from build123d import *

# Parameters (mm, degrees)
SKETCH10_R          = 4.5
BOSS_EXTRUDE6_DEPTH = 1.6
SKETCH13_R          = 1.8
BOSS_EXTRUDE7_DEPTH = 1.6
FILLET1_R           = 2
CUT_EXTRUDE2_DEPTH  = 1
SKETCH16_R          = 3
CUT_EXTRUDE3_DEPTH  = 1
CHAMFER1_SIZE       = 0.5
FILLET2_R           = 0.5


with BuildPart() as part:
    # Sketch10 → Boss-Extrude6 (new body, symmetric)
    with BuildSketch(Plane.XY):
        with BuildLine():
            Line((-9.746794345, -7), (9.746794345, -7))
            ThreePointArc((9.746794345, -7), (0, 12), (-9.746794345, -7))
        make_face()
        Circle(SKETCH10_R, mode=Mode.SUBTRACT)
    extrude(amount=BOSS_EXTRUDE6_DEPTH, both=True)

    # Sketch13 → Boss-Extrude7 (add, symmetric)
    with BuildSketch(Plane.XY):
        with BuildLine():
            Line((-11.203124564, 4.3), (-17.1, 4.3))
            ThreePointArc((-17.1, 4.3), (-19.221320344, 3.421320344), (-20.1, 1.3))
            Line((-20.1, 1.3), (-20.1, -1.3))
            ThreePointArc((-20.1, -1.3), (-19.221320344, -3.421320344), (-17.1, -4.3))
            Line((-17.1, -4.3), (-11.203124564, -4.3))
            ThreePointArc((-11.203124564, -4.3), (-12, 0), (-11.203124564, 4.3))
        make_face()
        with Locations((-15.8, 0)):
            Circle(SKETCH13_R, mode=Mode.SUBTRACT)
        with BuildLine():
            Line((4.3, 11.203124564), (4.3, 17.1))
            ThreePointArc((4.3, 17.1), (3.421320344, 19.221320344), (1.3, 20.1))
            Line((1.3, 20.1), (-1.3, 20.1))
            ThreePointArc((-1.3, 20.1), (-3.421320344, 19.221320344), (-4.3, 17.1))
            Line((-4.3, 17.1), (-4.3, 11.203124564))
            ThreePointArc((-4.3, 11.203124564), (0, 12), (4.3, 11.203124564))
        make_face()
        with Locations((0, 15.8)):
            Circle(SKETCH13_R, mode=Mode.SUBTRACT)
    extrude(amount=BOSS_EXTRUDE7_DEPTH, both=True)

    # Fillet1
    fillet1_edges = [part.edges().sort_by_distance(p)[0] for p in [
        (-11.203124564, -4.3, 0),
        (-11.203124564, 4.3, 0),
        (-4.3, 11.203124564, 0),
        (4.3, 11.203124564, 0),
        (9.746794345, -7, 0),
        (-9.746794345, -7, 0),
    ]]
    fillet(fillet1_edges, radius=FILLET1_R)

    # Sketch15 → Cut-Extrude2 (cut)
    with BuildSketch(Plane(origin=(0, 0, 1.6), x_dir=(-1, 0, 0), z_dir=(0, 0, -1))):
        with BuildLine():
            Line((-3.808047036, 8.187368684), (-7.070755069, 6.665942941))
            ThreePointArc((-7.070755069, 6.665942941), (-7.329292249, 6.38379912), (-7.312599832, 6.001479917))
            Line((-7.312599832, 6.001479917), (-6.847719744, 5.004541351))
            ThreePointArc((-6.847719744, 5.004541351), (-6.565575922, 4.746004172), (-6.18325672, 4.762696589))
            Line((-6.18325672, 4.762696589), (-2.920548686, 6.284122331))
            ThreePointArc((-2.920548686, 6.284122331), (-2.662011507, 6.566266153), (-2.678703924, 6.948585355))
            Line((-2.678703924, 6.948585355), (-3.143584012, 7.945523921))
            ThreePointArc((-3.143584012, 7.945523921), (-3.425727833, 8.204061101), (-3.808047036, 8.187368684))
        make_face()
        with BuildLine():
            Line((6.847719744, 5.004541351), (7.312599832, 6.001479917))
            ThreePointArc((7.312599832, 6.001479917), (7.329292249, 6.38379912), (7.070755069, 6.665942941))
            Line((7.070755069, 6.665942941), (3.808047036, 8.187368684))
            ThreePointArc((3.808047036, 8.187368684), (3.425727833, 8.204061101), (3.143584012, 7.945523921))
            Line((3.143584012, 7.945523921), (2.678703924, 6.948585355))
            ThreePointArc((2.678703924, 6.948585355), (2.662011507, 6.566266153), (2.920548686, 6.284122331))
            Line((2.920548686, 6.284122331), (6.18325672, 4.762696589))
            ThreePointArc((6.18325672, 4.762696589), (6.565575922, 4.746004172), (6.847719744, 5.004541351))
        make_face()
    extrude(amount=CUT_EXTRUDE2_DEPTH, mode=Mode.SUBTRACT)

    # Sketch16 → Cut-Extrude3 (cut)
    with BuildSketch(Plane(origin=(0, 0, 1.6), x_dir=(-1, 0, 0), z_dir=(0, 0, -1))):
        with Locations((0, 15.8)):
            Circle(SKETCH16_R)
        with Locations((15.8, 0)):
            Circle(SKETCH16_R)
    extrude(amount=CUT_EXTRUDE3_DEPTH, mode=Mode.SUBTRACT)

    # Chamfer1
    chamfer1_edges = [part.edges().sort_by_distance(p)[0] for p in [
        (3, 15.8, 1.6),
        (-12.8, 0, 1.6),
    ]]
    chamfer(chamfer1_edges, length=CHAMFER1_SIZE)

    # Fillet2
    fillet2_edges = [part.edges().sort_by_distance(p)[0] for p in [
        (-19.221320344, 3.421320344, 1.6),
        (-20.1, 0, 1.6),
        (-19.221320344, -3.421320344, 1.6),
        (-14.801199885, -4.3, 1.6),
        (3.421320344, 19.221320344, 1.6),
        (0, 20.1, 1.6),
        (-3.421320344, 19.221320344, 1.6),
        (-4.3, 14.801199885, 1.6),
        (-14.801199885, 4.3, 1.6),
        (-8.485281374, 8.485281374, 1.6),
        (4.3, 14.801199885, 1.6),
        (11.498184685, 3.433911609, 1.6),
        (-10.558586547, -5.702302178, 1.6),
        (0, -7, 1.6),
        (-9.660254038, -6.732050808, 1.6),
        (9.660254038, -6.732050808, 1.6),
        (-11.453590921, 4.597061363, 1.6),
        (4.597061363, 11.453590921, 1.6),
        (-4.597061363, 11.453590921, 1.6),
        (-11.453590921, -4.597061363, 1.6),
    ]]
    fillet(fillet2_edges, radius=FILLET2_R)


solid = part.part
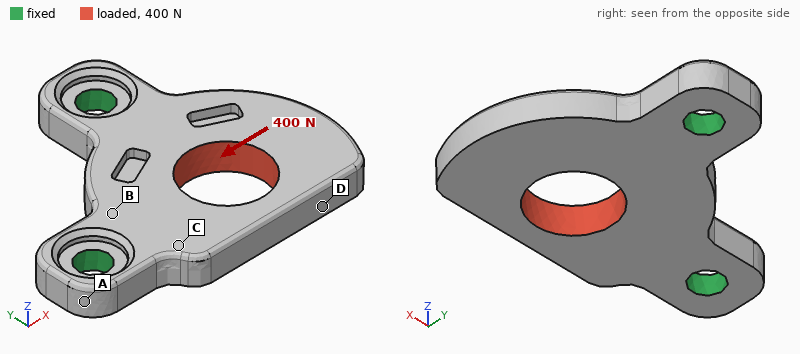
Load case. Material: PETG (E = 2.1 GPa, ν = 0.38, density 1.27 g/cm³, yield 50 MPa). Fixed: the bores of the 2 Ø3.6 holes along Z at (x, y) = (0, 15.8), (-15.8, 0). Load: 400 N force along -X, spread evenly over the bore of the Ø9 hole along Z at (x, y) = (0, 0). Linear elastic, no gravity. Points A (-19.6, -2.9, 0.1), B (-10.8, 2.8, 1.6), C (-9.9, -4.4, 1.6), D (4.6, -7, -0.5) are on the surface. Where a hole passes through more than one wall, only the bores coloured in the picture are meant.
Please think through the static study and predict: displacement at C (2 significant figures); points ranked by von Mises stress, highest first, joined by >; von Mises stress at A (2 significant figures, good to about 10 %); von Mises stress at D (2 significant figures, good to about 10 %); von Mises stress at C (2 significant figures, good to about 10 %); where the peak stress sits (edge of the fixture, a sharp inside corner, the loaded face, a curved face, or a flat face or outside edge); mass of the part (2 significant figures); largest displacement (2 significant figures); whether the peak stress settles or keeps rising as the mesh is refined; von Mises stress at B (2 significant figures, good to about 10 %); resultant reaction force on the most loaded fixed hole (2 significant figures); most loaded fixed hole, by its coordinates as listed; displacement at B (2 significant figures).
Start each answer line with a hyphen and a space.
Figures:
- 0.087 mm
- C > D > B > A
- 2.9 MPa
- 10 MPa
- 13 MPa
- edge of the fixture
- 1.7 g
- 0.22 mm
- keeps rising
- 6.1 MPa
- 340 N
- (-15.8, 0)
- 0.043 mm
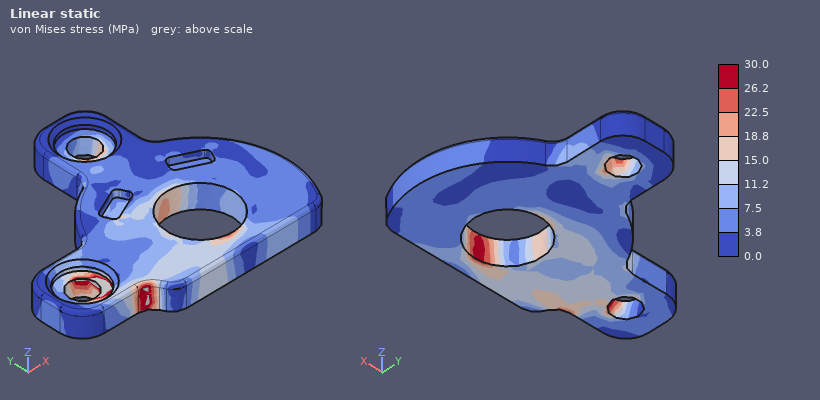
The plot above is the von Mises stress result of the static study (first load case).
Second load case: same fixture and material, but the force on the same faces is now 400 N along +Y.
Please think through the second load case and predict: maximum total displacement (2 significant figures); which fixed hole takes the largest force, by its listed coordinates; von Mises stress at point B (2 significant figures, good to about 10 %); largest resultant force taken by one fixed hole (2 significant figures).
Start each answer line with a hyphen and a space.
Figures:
- 0.23 mm
- (0, 15.8)
- 8.6 MPa
- 340 N
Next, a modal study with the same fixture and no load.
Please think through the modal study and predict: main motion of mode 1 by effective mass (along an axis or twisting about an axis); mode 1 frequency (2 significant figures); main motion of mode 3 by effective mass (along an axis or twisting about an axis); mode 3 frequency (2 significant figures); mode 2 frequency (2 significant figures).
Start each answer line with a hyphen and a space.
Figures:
- along Z
- 1400 Hz
- along Z
- 6400 Hz
- 4400 Hz
